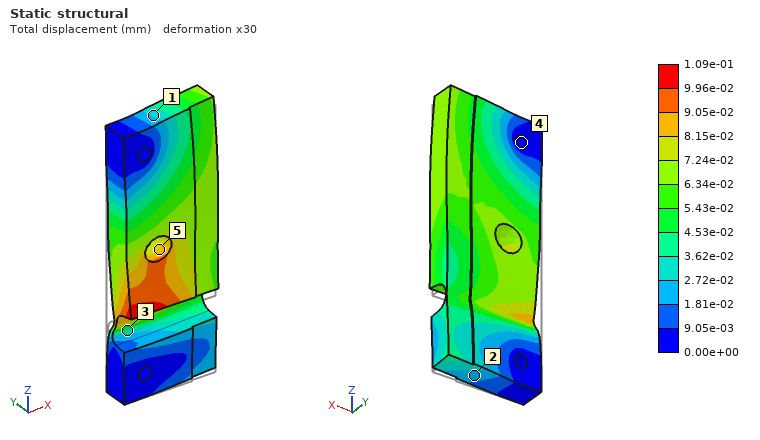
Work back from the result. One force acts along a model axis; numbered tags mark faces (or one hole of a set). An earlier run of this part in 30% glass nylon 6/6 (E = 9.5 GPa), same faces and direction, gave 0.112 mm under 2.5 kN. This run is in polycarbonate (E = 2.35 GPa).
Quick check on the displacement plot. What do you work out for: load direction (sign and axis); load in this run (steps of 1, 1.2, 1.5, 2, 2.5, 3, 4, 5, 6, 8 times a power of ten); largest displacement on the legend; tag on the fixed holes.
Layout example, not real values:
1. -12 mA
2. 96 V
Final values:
1. +Z
2. 600 N
3. 1.09e-01 mm
4. 4
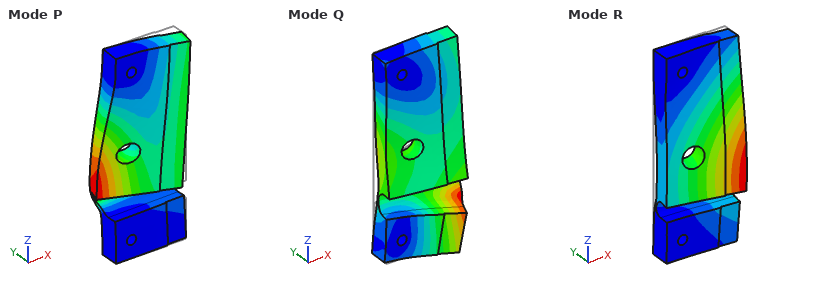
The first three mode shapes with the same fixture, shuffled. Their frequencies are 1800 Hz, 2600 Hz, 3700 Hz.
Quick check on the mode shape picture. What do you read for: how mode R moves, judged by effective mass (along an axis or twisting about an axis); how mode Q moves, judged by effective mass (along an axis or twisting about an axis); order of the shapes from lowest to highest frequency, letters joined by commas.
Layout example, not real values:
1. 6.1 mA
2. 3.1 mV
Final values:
1. along Y
2. along X
3. R, P, Q
